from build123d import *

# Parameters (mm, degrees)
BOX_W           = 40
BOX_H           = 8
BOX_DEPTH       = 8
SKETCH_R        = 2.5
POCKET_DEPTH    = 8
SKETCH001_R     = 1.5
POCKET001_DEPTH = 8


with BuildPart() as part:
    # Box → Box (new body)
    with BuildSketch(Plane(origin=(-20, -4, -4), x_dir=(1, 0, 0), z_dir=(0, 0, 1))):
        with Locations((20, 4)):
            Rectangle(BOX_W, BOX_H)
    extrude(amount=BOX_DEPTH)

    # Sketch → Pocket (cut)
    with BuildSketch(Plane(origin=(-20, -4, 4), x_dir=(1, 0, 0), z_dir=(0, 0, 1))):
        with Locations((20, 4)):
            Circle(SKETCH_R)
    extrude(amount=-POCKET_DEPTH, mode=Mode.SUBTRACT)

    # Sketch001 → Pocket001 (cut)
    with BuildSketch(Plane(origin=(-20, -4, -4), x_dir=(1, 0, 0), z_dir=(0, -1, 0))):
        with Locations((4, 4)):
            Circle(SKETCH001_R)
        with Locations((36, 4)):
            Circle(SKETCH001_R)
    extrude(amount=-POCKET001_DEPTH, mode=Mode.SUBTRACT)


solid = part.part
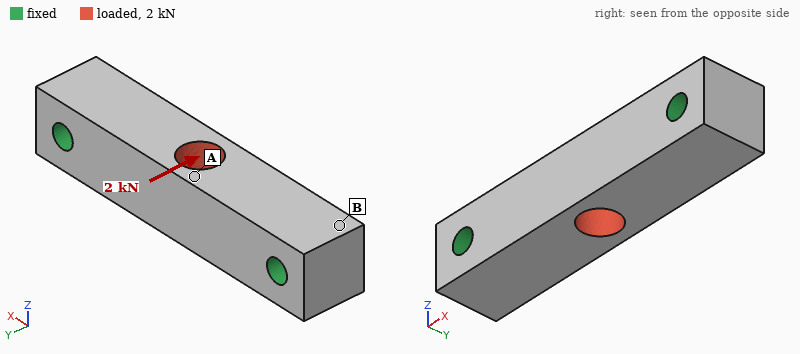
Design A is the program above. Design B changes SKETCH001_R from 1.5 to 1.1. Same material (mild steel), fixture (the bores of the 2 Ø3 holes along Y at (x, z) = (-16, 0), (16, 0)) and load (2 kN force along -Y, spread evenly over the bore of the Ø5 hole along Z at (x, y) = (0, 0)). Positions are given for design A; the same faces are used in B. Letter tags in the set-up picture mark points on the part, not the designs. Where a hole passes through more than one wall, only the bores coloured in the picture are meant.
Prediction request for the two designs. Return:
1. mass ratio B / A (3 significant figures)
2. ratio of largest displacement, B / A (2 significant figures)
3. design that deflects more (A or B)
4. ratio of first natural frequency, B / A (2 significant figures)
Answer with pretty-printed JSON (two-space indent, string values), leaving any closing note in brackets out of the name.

{
  "mass ratio B / A": "1.02",
  "ratio of largest displacement, B / A": "1.1",
  "design that deflects more": "B",
  "ratio of first natural frequency, B / A": "0.87"
}
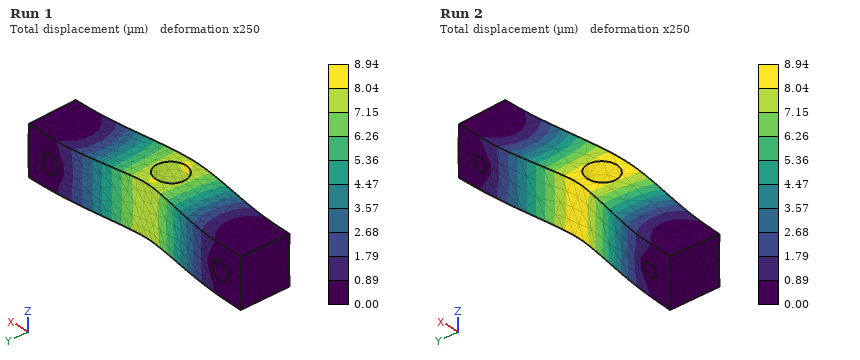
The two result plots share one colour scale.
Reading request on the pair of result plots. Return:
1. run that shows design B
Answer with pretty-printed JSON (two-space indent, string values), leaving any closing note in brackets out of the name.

{
  "run that shows design B": "Run 2"
}
